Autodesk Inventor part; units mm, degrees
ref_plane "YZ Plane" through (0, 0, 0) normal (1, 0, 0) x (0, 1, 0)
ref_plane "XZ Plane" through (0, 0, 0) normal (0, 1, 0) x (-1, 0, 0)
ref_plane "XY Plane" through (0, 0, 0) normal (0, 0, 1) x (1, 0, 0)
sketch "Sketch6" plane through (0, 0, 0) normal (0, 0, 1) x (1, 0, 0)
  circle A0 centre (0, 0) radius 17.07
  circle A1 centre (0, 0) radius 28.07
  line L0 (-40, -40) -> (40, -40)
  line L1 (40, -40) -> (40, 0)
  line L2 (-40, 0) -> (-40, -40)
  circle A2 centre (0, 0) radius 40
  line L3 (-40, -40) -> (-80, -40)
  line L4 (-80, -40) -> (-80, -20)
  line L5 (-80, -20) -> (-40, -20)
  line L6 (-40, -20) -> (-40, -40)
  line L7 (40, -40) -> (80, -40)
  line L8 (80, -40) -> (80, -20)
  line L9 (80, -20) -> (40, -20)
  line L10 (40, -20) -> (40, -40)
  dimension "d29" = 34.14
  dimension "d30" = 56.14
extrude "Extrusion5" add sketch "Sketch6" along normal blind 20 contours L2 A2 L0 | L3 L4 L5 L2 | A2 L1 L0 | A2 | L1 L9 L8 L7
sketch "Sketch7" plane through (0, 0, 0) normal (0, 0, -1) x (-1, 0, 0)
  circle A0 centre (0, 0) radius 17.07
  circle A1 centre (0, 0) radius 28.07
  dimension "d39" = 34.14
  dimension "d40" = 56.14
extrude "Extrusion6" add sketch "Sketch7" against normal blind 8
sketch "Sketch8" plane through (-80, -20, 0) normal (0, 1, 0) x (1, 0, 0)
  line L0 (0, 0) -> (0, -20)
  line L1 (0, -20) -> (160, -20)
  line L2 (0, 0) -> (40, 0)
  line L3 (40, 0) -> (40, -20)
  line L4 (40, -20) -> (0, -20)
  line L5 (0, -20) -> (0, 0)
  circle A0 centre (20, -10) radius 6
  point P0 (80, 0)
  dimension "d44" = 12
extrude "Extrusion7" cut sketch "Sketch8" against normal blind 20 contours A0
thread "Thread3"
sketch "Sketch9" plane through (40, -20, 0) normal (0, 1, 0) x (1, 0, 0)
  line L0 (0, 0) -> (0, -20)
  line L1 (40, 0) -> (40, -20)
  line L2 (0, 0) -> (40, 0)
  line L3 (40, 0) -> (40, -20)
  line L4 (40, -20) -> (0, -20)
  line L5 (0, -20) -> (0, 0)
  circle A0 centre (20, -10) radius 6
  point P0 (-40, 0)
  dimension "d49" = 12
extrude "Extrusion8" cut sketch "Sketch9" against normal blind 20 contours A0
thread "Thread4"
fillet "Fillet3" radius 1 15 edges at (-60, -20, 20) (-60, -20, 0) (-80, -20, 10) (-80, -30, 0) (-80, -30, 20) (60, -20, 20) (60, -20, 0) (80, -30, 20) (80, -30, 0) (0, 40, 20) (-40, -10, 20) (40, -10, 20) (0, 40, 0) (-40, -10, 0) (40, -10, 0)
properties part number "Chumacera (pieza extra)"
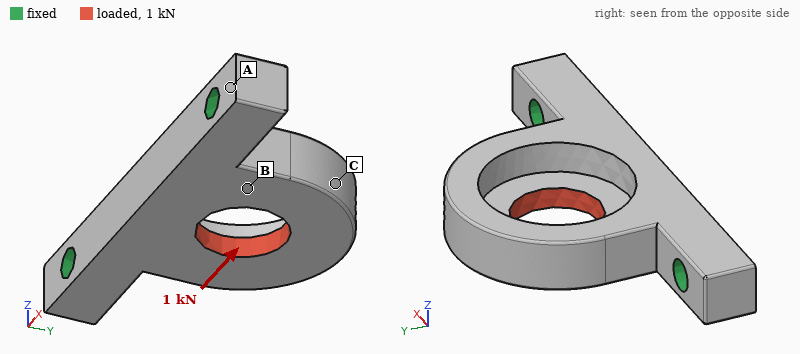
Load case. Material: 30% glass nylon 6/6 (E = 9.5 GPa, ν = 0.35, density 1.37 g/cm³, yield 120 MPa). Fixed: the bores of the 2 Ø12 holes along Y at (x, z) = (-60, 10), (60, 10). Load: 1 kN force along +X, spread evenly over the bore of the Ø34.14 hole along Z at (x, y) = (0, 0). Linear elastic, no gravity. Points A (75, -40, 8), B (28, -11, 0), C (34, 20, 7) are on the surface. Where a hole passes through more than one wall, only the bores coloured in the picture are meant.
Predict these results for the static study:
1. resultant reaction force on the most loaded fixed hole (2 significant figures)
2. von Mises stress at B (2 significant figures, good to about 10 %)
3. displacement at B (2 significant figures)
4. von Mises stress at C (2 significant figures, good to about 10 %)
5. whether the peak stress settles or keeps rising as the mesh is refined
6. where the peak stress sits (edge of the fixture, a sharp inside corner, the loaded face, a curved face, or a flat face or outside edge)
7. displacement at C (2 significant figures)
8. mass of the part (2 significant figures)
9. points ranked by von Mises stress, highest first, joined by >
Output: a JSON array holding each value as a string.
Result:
["590 N", "2.8 MPa", "12 µm", "1.5 MPa", "keeps rising", "a sharp inside corner", "35 µm", "140 g", "B > C > A"]
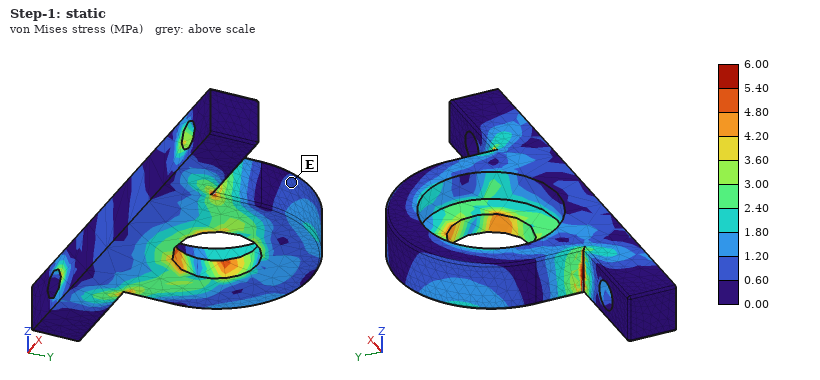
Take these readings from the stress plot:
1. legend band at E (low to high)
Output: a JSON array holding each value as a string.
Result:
["0.60 to 1.20 MPa"]
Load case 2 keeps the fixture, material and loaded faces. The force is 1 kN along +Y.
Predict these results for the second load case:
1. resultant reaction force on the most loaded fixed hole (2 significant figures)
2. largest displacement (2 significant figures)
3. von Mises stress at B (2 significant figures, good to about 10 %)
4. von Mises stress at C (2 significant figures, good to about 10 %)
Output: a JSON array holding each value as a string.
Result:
["520 N", "100 µm", "2.1 MPa", "1.0 MPa"]
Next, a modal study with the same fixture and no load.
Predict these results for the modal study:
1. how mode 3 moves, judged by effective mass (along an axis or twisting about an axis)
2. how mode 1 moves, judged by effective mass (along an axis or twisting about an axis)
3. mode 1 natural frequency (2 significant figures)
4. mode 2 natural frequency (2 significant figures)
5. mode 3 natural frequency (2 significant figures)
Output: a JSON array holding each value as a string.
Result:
["along X", "along Z", "960 Hz", "2500 Hz", "3300 Hz"]
